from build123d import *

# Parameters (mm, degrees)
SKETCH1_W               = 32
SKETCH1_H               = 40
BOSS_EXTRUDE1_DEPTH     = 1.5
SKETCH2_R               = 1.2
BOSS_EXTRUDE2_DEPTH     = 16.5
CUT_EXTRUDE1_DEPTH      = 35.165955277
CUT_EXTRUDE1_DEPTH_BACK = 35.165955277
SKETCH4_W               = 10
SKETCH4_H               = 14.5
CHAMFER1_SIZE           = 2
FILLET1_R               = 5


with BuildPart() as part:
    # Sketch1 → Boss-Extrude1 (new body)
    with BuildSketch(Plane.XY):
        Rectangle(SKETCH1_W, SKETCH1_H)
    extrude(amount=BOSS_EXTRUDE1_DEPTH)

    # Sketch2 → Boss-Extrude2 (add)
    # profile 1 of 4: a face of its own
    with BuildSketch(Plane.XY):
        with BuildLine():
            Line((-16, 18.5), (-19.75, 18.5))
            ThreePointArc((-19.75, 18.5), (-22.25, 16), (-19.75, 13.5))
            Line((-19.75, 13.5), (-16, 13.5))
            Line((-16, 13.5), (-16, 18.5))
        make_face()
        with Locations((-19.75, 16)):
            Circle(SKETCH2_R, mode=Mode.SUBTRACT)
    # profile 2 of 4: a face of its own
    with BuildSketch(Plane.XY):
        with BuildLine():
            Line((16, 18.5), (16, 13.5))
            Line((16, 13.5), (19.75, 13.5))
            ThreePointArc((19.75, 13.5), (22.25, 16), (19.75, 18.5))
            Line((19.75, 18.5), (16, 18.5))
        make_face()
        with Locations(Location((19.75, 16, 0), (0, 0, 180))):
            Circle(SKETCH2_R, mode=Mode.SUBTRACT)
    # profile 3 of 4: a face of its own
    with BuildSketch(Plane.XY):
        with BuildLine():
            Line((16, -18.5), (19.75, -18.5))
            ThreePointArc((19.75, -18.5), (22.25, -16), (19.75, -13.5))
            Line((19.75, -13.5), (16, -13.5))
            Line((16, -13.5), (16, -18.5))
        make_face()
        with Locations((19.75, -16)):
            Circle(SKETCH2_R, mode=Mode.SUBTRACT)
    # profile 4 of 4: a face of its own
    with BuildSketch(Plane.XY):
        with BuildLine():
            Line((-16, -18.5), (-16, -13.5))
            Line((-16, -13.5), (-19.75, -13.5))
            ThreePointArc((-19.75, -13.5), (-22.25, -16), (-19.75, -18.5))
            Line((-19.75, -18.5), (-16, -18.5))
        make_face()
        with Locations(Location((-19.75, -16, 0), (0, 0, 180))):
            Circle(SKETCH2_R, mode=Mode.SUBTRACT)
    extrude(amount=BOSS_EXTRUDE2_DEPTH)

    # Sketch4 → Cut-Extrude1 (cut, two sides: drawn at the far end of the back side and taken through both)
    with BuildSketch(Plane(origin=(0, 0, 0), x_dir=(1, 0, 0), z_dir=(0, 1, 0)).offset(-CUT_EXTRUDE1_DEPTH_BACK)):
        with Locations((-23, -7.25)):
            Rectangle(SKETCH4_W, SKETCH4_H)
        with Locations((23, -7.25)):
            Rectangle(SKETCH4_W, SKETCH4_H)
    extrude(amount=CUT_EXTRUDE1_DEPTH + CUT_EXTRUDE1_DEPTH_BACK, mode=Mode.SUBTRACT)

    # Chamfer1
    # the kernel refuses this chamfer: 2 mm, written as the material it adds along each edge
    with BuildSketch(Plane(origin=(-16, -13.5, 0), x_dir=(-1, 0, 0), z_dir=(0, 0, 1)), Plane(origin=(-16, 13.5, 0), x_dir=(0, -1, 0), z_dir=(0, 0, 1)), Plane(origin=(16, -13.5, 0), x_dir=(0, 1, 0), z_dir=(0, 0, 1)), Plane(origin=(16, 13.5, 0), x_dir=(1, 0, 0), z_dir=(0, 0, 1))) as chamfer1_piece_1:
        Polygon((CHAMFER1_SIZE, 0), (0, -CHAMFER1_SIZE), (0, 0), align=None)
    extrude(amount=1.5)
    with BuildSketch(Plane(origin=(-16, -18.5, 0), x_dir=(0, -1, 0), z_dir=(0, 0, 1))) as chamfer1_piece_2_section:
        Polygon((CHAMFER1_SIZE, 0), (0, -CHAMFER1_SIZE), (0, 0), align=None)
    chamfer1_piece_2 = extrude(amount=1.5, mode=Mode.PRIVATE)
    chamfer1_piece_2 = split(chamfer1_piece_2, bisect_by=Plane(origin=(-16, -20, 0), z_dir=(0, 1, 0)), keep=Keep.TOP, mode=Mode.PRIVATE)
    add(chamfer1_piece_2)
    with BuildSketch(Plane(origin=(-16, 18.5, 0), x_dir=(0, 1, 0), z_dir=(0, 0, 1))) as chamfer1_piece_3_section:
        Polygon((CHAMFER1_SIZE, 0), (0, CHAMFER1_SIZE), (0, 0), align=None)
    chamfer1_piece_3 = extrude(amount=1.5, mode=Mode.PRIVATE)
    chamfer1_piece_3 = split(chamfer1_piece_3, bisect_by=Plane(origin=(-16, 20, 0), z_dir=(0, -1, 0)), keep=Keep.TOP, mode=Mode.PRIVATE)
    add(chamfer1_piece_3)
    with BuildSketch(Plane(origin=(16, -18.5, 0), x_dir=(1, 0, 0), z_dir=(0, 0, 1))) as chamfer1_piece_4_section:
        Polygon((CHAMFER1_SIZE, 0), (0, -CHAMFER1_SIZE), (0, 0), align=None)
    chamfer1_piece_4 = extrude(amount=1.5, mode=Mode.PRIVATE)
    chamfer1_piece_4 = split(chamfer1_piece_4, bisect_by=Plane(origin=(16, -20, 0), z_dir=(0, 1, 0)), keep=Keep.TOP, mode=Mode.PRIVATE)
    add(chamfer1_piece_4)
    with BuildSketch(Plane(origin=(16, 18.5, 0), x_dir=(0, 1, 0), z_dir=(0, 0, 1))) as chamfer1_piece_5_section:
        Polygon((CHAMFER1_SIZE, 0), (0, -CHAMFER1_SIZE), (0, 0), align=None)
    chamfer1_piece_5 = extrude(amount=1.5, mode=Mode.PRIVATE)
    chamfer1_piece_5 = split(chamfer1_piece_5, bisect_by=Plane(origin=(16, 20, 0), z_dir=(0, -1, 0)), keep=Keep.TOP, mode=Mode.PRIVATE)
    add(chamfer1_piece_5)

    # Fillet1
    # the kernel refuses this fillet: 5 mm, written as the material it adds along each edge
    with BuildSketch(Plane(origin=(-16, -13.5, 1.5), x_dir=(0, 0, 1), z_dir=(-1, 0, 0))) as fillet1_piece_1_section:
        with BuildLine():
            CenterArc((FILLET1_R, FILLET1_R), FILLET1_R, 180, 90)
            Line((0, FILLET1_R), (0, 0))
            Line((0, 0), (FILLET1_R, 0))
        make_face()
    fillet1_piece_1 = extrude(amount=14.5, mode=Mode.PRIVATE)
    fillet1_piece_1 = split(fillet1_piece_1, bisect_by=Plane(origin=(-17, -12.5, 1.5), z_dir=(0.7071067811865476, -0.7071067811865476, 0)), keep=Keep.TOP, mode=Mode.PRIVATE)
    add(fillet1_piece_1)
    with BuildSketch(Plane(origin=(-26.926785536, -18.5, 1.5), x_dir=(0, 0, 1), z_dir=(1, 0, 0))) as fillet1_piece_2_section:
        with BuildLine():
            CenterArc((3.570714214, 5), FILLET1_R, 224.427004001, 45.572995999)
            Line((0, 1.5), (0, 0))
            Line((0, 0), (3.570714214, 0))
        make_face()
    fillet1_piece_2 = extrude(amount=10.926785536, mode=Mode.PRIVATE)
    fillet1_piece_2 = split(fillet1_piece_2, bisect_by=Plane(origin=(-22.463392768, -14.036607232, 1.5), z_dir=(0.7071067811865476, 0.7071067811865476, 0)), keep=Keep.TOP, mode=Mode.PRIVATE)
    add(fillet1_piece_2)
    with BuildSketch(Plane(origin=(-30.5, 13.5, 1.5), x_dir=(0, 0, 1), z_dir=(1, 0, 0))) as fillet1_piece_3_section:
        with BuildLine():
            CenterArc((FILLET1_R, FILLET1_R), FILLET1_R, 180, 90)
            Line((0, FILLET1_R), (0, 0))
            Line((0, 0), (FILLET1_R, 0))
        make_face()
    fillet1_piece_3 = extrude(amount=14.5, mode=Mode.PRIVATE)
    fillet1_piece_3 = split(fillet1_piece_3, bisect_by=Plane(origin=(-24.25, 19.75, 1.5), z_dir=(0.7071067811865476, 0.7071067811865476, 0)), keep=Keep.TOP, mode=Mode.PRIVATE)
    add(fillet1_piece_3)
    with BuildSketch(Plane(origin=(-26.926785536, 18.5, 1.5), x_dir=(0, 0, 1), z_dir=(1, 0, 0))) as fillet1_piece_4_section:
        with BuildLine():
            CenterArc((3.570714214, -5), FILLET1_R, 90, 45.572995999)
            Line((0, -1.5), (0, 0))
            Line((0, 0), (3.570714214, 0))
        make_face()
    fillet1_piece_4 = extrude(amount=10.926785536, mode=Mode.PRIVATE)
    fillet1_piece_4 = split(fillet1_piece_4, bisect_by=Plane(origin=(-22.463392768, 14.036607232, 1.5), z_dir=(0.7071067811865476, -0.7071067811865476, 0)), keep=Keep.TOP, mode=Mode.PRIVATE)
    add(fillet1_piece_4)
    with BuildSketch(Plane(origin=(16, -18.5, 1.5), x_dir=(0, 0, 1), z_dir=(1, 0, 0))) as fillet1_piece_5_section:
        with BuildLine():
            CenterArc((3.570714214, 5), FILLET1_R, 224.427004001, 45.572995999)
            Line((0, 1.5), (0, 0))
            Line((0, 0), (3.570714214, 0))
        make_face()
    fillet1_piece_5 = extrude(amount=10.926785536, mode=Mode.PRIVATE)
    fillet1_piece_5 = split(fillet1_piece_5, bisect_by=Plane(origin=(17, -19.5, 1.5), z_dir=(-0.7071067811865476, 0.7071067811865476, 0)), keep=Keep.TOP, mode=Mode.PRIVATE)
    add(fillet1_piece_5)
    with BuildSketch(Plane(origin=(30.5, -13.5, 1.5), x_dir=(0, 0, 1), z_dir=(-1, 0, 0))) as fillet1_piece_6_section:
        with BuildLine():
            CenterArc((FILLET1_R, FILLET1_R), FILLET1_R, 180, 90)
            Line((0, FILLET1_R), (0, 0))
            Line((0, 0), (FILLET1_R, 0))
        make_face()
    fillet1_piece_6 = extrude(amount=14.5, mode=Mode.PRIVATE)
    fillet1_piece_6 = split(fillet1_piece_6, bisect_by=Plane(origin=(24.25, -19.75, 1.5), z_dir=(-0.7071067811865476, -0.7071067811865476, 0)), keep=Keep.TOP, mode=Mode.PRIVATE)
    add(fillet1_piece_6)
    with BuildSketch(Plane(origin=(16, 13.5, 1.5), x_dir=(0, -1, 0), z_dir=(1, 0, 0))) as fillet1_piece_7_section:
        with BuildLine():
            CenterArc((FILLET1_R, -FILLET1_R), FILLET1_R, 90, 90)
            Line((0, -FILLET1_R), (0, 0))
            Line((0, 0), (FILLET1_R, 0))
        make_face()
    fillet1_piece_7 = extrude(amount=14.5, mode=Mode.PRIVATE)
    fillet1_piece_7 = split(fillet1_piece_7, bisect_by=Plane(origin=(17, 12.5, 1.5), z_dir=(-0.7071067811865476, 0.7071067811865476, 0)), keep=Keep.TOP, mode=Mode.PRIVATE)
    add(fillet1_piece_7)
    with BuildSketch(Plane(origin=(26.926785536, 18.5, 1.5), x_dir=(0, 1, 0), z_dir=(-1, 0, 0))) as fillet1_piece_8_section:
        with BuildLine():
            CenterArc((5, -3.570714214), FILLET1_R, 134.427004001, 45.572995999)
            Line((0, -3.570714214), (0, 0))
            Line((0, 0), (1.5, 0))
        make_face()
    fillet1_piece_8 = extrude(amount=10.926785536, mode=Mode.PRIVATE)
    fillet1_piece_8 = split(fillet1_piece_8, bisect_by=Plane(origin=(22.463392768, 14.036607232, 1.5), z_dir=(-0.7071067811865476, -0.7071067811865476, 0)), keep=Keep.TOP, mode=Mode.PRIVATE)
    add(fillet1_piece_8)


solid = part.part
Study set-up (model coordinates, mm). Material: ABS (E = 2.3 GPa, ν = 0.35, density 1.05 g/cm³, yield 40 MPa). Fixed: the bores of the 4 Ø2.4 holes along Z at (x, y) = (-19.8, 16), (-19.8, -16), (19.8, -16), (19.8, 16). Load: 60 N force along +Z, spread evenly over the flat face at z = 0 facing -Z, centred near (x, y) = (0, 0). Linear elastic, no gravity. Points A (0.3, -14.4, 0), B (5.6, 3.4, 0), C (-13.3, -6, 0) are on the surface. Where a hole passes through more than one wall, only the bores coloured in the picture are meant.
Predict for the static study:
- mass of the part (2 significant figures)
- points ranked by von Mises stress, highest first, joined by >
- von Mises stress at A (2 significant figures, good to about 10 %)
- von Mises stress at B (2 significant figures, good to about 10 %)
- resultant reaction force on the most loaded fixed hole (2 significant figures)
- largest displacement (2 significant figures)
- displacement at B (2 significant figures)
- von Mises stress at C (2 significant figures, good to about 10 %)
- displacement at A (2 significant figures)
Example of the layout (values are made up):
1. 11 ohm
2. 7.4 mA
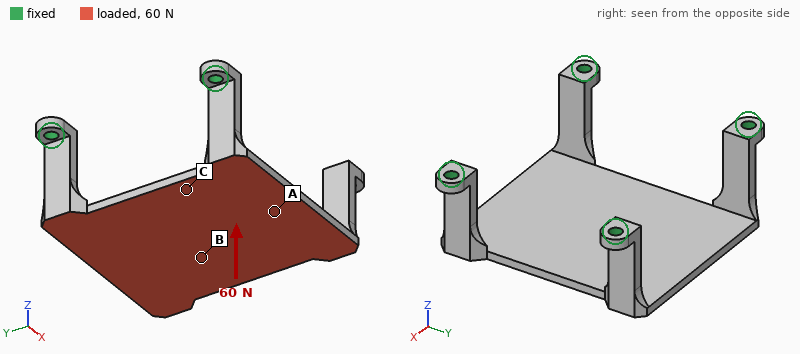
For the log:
1. 2.9 g
2. A > B > C
3. 9.0 MPa
4. 7.1 MPa
5. 17 N
6. 0.64 mm
7. 0.57 mm
8. 5.0 MPa
9. 0.51 mm
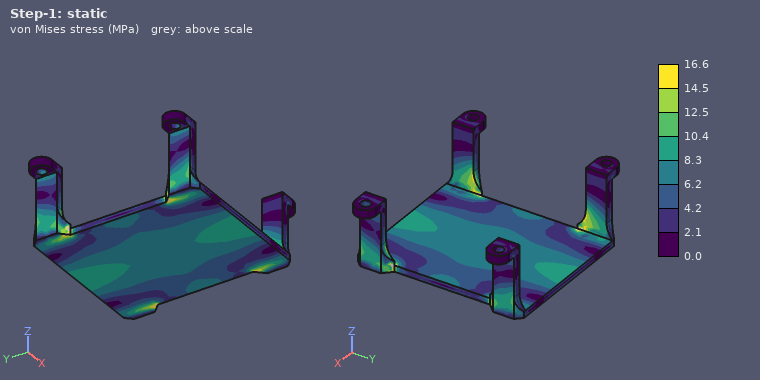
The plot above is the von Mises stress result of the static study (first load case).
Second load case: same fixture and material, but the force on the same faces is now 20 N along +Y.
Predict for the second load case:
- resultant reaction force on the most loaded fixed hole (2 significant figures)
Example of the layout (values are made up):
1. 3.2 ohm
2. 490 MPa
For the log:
1. 5.2 N
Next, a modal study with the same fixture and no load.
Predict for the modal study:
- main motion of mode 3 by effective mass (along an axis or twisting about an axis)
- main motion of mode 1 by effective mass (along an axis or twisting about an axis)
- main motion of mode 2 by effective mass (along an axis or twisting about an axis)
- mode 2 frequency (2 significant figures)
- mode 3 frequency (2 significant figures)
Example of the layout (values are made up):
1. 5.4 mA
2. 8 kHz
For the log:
1. along Z
2. along X
3. along Y
4. 1100 Hz
5. 1300 Hz
